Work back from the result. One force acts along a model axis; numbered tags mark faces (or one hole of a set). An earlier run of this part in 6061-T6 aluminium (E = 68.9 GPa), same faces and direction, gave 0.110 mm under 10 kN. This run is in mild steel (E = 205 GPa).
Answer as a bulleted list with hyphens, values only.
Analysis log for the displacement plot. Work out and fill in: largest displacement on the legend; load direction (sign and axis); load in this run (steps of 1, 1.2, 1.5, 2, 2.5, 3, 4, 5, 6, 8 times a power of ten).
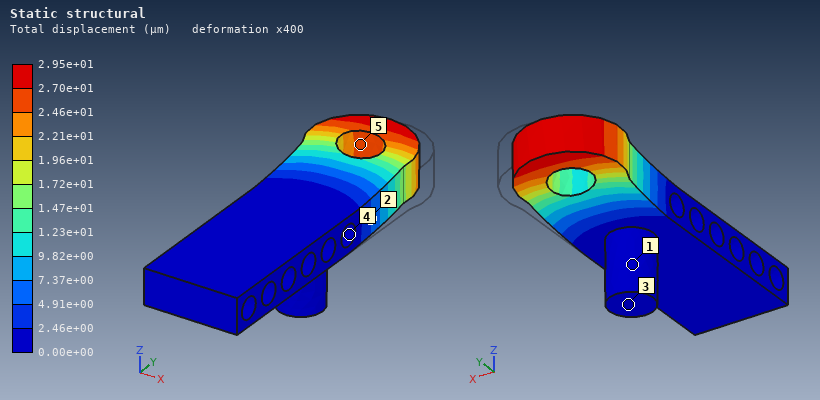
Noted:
- 2.95e+01 µm
- -X
- 8 kN
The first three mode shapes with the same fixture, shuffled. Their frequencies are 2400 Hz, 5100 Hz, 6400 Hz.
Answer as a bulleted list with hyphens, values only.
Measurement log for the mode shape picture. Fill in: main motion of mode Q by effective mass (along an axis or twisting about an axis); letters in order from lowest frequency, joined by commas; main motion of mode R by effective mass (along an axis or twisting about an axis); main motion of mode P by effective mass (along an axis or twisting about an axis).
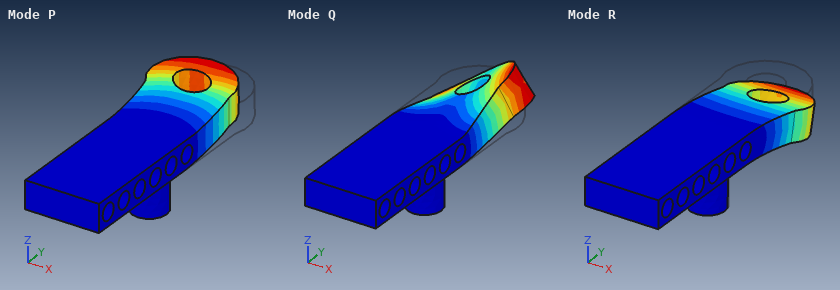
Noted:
- twisting about Y
- R, P, Q
- along Z
- along X
